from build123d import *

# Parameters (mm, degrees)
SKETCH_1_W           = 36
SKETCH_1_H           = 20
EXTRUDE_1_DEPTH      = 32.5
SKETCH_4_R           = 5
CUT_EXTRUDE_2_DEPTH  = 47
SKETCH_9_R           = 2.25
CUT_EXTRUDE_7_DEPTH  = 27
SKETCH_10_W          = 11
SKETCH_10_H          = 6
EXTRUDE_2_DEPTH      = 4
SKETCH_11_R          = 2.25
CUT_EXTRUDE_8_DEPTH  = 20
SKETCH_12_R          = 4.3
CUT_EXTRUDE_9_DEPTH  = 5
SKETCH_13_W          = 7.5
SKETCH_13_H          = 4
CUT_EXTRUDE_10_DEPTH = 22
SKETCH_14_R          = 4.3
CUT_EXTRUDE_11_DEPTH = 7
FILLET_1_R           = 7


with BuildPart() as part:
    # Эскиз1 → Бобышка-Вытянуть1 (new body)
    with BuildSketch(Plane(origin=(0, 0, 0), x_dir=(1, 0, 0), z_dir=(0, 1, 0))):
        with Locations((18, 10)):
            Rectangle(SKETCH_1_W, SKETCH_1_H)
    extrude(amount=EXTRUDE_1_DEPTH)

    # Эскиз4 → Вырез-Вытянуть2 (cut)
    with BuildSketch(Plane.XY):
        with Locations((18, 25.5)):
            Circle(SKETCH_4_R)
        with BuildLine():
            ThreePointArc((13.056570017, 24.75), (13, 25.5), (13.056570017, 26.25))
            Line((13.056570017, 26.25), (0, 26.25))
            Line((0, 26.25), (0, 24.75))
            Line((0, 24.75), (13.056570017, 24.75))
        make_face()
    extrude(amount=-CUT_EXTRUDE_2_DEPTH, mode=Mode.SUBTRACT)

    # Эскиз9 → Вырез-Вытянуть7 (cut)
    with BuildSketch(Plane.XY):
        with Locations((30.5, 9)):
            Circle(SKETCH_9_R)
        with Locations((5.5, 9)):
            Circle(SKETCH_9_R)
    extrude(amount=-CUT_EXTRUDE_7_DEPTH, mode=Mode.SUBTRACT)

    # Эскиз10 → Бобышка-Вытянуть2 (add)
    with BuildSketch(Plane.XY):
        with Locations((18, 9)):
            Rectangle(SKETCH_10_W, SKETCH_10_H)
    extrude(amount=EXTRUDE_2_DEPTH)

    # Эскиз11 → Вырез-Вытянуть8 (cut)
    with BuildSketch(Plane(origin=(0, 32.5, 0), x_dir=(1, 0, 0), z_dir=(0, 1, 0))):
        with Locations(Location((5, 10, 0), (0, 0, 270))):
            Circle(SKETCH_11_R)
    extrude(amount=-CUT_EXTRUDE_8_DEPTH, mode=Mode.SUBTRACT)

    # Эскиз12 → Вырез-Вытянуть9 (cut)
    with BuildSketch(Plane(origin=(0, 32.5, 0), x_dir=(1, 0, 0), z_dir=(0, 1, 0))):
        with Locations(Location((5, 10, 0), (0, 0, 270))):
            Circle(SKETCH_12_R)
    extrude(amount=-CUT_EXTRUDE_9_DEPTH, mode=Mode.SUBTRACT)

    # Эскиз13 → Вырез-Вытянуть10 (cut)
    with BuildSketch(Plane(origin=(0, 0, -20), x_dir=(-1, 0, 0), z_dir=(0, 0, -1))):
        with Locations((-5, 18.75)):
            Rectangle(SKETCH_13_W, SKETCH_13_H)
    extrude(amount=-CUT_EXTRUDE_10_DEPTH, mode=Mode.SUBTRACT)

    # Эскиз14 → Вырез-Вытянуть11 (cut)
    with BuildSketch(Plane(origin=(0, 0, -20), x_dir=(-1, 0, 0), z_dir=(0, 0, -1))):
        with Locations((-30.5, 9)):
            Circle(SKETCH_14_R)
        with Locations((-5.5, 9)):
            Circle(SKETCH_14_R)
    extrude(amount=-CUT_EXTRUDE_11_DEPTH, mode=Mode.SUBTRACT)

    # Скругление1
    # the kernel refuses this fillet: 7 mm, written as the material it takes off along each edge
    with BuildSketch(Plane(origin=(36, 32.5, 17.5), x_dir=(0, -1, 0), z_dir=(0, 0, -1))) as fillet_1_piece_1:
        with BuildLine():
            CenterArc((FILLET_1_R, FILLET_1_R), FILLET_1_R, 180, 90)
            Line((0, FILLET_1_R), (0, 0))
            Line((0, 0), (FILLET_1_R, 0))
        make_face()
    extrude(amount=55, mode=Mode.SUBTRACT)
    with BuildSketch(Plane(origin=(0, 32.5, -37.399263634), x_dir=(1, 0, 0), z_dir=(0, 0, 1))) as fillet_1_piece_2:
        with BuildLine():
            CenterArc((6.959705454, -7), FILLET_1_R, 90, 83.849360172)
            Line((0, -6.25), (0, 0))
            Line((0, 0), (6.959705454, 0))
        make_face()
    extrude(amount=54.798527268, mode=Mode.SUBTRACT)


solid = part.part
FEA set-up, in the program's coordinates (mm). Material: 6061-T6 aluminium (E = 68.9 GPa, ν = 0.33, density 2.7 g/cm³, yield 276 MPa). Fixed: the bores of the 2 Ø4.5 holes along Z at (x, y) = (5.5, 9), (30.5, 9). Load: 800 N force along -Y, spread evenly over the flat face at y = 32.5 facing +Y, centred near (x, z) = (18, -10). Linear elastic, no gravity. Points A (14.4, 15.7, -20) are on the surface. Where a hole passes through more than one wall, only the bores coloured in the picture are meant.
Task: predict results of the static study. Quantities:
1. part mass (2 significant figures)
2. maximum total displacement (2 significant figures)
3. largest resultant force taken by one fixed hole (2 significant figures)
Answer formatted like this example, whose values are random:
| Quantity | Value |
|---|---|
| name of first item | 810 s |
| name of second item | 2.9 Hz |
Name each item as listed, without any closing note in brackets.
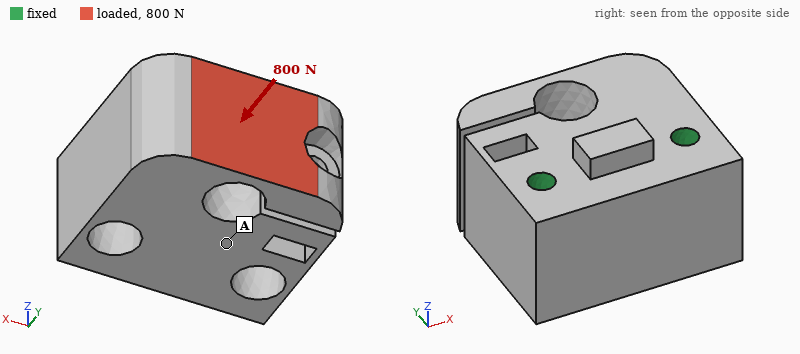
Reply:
| Quantity | Value |
|---|---|
| part mass | 51 g |
| maximum total displacement | 0.26 mm |
| largest resultant force taken by one fixed hole | 450 N |
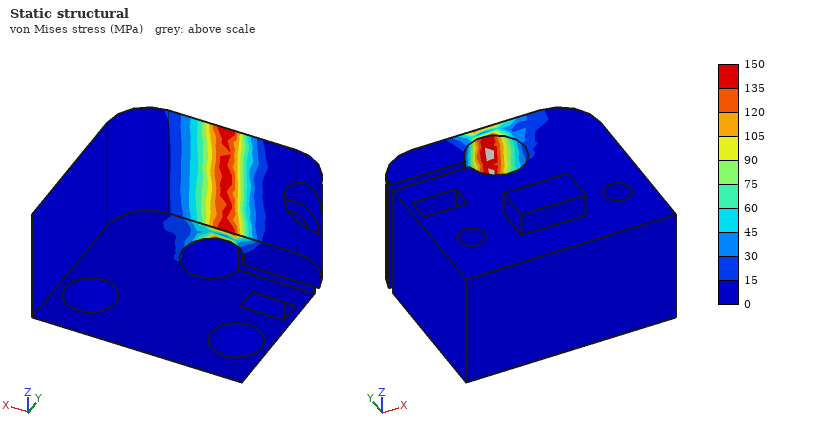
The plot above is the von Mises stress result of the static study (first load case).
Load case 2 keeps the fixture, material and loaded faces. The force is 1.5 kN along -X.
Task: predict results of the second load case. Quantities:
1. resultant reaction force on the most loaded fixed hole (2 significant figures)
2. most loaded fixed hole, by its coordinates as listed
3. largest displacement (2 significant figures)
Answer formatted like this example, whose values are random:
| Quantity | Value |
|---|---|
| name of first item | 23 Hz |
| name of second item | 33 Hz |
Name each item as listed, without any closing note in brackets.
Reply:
| Quantity | Value |
|---|---|
| resultant reaction force on the most loaded fixed hole | 1.6 kN |
| most loaded fixed hole, by its coordinates as listed | (5.5, 9) |
| largest displacement | 0.13 mm |
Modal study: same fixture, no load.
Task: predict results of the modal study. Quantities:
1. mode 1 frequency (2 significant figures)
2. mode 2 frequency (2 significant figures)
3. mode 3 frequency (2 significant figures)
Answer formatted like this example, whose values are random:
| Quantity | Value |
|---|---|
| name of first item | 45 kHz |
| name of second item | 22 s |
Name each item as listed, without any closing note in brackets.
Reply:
| Quantity | Value |
|---|---|
| mode 1 frequency | 3200 Hz |
| mode 2 frequency | 8700 Hz |
| mode 3 frequency | 11 kHz |
